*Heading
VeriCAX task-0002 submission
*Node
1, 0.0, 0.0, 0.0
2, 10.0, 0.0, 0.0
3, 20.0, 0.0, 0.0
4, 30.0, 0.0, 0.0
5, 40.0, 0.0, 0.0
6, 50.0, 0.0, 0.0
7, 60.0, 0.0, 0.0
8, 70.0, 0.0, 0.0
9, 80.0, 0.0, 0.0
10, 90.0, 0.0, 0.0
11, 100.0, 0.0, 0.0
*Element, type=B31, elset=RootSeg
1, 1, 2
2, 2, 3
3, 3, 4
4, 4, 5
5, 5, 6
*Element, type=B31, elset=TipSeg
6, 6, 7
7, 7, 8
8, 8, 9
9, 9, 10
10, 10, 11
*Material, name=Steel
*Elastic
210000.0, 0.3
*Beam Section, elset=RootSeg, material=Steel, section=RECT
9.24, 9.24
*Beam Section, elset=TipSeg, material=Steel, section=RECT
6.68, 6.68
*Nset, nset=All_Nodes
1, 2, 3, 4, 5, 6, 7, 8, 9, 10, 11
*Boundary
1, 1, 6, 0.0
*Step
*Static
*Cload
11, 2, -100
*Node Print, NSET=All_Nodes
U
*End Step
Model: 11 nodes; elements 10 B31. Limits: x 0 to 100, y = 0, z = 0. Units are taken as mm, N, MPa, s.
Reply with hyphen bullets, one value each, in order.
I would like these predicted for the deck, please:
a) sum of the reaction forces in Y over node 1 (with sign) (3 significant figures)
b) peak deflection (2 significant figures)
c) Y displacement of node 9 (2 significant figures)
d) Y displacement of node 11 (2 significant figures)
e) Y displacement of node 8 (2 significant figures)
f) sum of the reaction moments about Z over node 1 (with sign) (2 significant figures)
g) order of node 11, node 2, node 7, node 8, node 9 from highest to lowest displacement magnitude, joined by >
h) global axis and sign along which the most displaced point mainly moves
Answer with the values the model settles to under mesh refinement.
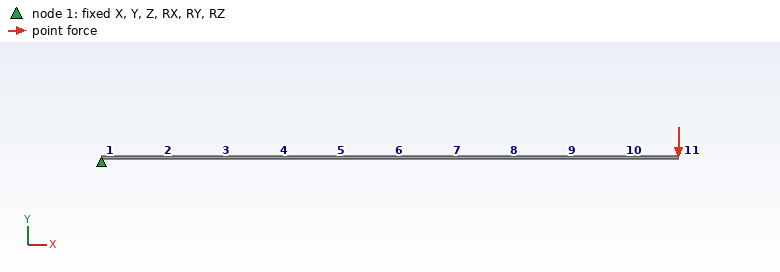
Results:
- 100 N
- 0.35 mm
- -0.22 mm
- -0.35 mm
- -0.17 mm
- 10000 N·mm
- node 11 > node 9 > node 8 > node 7 > node 2
- -Y
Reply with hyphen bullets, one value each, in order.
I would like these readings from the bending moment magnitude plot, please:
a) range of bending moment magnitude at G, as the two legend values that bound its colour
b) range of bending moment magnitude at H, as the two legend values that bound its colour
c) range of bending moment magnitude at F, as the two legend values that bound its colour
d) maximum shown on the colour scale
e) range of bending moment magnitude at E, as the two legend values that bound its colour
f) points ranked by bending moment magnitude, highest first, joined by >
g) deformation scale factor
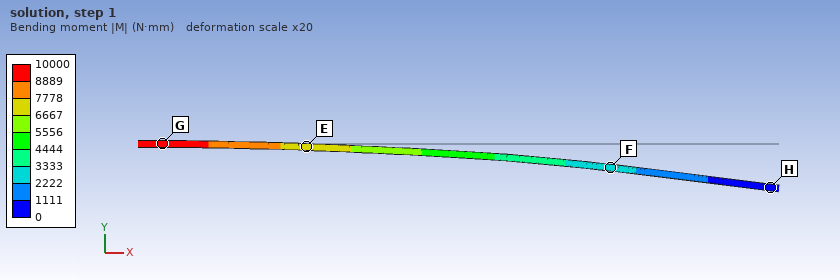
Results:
- 8889 to 10000 N·mm
- 0 to 1111 N·mm
- 2222 to 3333 N·mm
- 10000 N·mm
- 6667 to 7778 N·mm
- G > E > F > H
- 20
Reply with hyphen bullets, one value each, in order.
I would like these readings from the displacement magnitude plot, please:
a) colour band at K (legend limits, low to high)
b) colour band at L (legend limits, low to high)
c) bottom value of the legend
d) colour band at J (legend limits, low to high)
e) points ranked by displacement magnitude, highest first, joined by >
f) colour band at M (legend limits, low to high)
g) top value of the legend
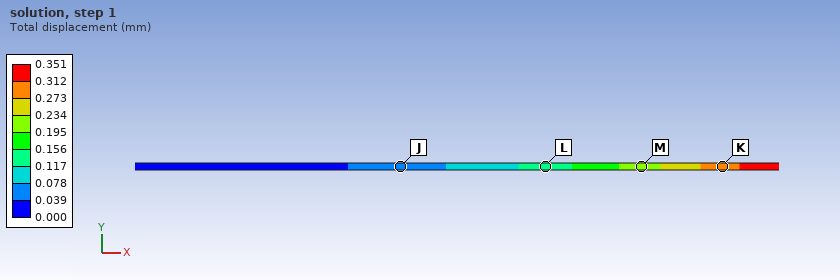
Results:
- 0.273 to 0.312 mm
- 0.117 to 0.156 mm
- 0.000 mm
- 0.039 to 0.078 mm
- K > M > L > J
- 0.195 to 0.234 mm
- 0.351 mm
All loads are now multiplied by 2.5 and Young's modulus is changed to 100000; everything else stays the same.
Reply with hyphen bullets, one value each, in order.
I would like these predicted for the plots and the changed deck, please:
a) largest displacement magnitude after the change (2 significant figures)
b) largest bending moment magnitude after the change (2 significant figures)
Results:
- 1.8 mm
- 25000 N·mm
